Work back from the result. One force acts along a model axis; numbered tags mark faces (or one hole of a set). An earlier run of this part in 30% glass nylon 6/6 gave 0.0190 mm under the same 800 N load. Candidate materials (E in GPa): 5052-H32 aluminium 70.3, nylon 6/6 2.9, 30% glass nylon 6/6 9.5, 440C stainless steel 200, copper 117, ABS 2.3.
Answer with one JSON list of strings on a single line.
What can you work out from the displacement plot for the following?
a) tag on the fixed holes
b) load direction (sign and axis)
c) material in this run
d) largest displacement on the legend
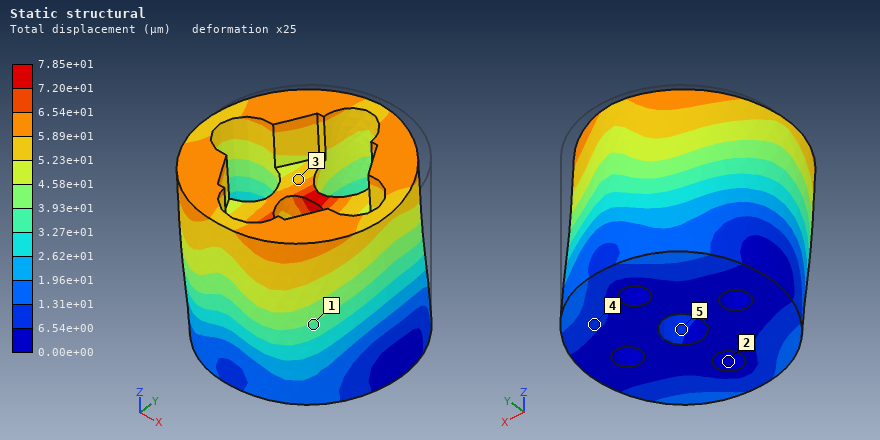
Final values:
["2", "-Y", "ABS", "7.85e+01 µm"]
